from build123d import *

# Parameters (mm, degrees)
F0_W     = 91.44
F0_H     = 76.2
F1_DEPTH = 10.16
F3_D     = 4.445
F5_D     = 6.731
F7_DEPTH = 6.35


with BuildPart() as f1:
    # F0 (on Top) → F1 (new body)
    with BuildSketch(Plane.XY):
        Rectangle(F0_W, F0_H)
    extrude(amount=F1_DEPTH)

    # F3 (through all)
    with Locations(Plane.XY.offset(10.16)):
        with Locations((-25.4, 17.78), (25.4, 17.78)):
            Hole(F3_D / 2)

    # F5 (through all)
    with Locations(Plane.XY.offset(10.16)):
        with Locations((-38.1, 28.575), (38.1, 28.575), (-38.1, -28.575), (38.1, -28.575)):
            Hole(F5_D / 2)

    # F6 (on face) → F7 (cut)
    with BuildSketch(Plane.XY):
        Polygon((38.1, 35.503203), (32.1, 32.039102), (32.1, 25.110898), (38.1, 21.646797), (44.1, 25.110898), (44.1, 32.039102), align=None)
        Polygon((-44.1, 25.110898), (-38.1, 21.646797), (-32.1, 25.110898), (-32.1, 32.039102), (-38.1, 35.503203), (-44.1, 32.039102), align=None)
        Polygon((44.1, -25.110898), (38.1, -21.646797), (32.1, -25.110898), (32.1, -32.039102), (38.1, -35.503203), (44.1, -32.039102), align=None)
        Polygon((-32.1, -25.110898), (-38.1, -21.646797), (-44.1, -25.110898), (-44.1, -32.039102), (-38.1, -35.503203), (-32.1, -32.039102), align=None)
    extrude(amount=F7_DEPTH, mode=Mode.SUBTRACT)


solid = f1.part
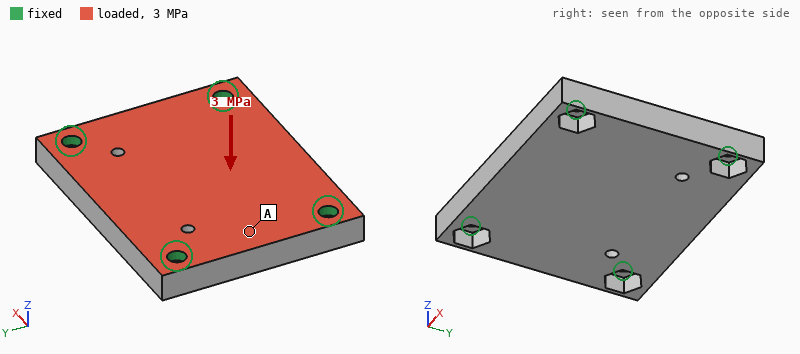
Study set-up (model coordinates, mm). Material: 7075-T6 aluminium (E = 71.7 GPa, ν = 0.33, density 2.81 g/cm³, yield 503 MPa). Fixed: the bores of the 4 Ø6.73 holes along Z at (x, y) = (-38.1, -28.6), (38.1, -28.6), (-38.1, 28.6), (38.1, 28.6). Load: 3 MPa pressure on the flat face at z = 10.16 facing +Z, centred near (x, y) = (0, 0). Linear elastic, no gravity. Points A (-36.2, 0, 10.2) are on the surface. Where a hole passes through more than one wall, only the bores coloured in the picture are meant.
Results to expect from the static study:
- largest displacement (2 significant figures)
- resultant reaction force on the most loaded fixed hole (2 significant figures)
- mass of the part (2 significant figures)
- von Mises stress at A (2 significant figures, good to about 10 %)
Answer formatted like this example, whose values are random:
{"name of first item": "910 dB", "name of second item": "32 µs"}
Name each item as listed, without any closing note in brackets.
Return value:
{"largest displacement": "0.12 mm", "resultant reaction force on the most loaded fixed hole": "6.8 kN", "mass of the part": "190 g", "von Mises stress at A": "31 MPa"}
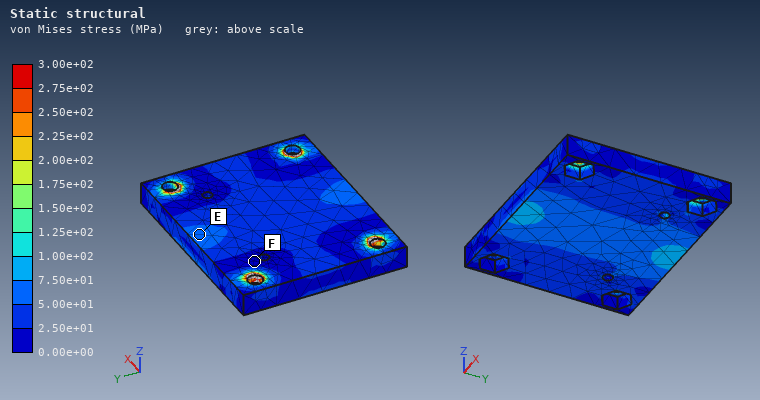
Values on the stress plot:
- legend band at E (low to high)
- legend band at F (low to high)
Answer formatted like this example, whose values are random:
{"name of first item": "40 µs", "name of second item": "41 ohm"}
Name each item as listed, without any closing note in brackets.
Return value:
{"legend band at E": "5.00e+01 to 7.50e+01 MPa", "legend band at F": "0.00e+00 to 2.50e+01 MPa"}
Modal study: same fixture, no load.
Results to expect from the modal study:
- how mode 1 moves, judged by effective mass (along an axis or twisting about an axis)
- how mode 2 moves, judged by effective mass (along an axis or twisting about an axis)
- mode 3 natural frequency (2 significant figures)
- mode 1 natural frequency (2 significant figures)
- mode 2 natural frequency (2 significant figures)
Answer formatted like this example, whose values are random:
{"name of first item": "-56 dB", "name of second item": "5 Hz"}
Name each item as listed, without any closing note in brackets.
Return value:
{"how mode 1 moves, judged by effective mass": "along Z", "how mode 2 moves, judged by effective mass": "twisting about X", "mode 3 natural frequency": "10 kHz", "mode 1 natural frequency": "5400 Hz", "mode 2 natural frequency": "7800 Hz"}
